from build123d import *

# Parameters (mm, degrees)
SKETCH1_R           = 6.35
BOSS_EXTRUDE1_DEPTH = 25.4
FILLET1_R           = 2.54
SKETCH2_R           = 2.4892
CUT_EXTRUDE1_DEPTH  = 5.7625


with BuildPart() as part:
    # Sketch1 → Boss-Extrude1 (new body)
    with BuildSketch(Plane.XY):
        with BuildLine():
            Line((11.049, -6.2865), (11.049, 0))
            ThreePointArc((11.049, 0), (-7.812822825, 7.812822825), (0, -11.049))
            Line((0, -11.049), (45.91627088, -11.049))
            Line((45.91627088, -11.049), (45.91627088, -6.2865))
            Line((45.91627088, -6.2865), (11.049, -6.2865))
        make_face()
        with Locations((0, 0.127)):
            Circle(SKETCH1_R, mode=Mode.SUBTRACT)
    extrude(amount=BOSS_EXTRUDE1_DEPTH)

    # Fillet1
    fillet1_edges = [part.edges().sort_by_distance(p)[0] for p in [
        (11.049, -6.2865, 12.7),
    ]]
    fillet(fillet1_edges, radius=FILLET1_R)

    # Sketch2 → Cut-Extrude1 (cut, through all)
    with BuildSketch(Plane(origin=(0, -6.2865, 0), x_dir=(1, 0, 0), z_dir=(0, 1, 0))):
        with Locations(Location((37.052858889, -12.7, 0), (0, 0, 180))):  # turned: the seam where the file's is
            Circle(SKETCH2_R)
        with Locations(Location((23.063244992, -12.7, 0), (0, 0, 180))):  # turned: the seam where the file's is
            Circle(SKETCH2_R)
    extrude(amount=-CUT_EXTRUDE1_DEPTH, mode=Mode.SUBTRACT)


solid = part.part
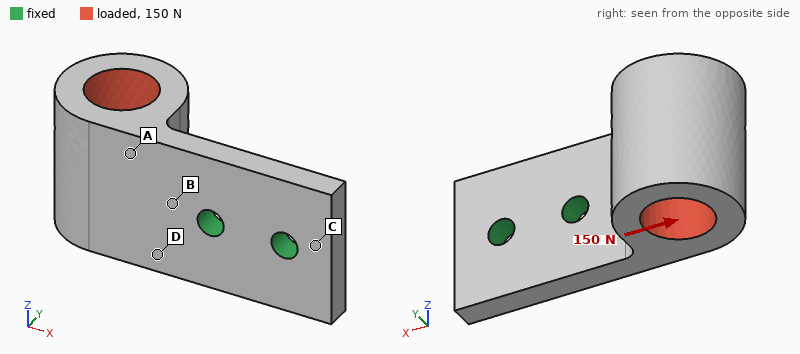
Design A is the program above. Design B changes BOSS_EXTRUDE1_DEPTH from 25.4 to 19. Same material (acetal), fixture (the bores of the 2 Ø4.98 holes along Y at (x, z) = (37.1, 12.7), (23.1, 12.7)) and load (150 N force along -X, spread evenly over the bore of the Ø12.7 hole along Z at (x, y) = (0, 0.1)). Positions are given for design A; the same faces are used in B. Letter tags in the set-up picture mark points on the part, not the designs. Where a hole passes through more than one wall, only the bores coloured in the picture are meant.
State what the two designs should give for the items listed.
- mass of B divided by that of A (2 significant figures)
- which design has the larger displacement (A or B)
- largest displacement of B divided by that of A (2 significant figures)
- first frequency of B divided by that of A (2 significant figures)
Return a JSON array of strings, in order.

["0.74", "B", "1.3", "1.0"]
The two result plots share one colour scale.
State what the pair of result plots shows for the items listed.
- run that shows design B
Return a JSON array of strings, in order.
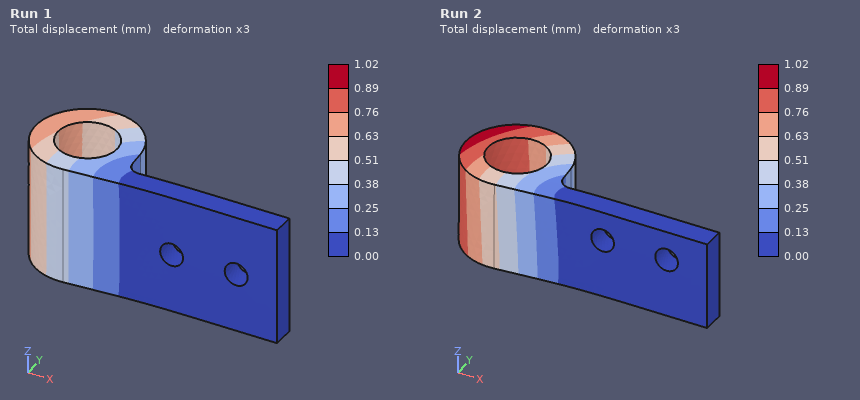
["Run 2"]
